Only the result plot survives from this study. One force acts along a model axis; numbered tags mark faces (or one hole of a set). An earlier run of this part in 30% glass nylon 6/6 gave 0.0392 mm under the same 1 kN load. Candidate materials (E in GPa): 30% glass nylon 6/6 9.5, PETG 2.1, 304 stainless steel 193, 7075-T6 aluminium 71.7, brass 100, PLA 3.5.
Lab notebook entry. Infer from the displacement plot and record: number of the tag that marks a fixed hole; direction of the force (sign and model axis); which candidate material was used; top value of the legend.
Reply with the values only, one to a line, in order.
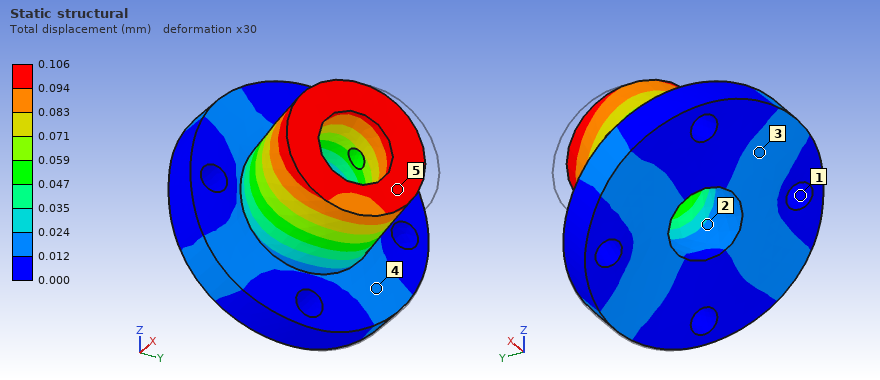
1
-Y
PLA
0.106 mm
